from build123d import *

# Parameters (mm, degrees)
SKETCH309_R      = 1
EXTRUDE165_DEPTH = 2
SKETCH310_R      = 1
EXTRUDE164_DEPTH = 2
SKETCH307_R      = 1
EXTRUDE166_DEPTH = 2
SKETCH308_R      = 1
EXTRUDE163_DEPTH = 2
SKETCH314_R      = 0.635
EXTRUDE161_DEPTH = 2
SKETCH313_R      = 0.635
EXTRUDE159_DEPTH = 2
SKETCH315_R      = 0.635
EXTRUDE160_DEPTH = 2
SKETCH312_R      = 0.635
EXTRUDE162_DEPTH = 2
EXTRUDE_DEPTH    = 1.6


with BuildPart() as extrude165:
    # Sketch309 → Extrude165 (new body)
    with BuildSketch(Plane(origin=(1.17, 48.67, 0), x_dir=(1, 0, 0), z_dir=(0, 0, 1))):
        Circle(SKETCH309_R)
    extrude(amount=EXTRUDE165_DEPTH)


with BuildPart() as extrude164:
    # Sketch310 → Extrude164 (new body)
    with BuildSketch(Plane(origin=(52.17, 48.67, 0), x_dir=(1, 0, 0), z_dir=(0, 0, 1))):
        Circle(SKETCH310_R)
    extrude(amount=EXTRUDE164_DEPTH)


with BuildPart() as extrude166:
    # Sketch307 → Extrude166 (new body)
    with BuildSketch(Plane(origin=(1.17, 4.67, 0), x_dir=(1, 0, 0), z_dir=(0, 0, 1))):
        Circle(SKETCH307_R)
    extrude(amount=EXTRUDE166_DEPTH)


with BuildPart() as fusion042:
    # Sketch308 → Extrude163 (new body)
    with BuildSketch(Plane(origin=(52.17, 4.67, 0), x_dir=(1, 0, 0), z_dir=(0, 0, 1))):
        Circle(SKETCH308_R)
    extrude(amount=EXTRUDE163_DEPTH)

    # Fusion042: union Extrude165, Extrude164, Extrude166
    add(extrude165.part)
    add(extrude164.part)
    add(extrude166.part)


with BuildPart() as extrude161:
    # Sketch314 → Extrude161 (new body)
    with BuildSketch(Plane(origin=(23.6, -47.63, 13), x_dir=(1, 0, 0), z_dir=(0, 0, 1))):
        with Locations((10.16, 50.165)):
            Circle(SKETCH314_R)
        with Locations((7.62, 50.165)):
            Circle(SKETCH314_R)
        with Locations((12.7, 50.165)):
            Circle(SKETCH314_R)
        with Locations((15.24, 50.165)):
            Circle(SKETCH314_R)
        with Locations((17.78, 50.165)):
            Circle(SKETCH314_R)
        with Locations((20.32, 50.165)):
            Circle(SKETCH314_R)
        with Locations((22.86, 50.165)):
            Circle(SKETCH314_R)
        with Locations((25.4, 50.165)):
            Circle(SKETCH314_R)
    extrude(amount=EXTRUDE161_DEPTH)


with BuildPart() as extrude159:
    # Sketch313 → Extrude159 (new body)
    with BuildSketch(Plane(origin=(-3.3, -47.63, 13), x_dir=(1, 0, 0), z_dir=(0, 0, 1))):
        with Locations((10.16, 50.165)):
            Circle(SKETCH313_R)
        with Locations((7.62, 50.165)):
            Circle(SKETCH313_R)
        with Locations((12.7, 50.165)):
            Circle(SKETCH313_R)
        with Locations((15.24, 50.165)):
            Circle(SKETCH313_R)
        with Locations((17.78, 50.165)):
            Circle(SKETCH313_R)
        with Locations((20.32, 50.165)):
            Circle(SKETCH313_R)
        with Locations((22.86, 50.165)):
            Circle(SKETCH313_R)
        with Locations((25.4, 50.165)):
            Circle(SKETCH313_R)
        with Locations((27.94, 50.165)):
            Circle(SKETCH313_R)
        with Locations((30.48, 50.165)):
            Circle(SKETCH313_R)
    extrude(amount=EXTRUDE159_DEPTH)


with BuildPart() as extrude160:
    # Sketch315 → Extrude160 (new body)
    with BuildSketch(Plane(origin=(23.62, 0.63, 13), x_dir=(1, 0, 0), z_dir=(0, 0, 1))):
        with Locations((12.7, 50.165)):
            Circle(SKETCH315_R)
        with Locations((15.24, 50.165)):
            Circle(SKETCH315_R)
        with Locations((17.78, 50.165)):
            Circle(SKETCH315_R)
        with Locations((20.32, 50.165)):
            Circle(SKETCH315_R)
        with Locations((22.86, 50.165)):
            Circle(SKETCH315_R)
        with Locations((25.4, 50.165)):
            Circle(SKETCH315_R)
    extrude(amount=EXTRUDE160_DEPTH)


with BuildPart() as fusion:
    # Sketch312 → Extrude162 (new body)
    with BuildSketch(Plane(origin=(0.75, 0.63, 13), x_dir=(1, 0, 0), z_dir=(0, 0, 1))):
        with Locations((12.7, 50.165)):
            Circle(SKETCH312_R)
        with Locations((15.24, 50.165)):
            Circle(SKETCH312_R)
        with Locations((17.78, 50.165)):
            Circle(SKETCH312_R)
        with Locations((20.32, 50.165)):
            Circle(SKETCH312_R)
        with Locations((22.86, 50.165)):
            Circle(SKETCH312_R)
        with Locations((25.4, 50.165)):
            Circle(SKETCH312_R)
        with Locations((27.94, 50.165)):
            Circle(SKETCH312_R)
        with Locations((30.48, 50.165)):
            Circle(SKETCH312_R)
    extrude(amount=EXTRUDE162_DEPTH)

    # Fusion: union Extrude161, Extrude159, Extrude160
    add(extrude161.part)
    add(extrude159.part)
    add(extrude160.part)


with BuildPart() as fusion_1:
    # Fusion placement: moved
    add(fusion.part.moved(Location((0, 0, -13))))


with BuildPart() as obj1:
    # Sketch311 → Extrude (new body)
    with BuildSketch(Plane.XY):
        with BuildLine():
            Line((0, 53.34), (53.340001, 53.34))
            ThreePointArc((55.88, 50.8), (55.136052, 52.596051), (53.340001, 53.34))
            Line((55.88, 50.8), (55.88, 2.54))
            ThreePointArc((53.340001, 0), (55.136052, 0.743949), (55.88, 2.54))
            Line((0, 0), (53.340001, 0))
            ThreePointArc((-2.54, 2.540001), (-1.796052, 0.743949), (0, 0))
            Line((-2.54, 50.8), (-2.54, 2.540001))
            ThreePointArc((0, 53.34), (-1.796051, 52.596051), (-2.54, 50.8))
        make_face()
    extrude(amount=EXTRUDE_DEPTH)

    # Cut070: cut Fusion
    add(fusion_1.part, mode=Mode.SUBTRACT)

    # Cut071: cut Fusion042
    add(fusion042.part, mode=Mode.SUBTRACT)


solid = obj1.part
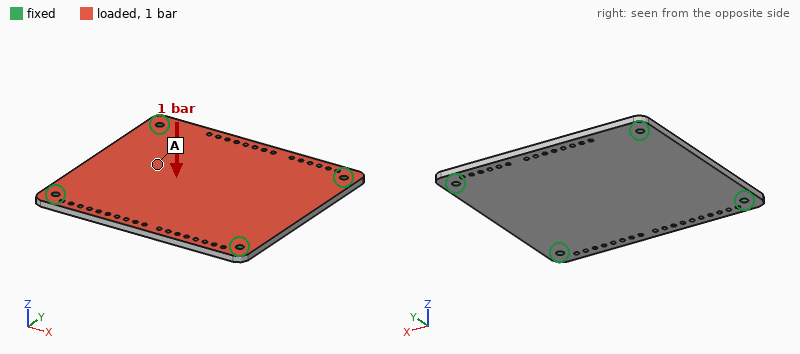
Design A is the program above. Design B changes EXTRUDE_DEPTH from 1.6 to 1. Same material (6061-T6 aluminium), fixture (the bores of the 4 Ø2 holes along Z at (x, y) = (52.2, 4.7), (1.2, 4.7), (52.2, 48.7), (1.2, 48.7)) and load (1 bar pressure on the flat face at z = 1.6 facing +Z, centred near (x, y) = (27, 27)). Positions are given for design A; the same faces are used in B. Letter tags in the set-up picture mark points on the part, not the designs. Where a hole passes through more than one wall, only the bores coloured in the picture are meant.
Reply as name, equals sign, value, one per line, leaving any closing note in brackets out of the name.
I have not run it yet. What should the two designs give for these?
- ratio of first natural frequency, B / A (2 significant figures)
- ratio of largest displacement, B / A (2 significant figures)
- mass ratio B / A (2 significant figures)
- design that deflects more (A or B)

ratio of first natural frequency, B / A = 0.64
ratio of largest displacement, B / A = 3.9
mass ratio B / A = 0.63
design that deflects more = B
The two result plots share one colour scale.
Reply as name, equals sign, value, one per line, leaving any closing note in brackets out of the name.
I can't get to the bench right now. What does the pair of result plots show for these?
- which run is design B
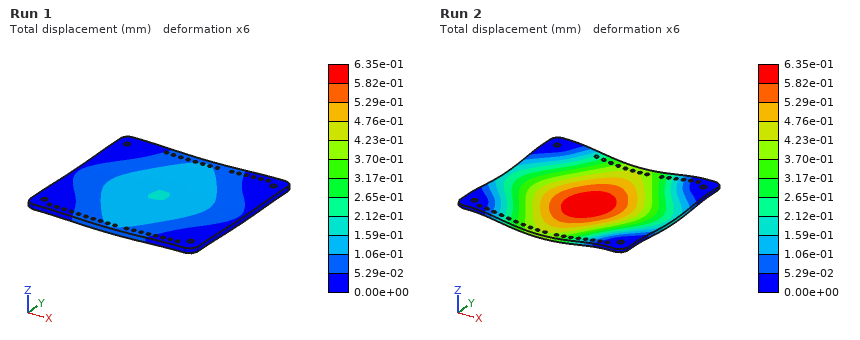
which run is design B = Run 2
